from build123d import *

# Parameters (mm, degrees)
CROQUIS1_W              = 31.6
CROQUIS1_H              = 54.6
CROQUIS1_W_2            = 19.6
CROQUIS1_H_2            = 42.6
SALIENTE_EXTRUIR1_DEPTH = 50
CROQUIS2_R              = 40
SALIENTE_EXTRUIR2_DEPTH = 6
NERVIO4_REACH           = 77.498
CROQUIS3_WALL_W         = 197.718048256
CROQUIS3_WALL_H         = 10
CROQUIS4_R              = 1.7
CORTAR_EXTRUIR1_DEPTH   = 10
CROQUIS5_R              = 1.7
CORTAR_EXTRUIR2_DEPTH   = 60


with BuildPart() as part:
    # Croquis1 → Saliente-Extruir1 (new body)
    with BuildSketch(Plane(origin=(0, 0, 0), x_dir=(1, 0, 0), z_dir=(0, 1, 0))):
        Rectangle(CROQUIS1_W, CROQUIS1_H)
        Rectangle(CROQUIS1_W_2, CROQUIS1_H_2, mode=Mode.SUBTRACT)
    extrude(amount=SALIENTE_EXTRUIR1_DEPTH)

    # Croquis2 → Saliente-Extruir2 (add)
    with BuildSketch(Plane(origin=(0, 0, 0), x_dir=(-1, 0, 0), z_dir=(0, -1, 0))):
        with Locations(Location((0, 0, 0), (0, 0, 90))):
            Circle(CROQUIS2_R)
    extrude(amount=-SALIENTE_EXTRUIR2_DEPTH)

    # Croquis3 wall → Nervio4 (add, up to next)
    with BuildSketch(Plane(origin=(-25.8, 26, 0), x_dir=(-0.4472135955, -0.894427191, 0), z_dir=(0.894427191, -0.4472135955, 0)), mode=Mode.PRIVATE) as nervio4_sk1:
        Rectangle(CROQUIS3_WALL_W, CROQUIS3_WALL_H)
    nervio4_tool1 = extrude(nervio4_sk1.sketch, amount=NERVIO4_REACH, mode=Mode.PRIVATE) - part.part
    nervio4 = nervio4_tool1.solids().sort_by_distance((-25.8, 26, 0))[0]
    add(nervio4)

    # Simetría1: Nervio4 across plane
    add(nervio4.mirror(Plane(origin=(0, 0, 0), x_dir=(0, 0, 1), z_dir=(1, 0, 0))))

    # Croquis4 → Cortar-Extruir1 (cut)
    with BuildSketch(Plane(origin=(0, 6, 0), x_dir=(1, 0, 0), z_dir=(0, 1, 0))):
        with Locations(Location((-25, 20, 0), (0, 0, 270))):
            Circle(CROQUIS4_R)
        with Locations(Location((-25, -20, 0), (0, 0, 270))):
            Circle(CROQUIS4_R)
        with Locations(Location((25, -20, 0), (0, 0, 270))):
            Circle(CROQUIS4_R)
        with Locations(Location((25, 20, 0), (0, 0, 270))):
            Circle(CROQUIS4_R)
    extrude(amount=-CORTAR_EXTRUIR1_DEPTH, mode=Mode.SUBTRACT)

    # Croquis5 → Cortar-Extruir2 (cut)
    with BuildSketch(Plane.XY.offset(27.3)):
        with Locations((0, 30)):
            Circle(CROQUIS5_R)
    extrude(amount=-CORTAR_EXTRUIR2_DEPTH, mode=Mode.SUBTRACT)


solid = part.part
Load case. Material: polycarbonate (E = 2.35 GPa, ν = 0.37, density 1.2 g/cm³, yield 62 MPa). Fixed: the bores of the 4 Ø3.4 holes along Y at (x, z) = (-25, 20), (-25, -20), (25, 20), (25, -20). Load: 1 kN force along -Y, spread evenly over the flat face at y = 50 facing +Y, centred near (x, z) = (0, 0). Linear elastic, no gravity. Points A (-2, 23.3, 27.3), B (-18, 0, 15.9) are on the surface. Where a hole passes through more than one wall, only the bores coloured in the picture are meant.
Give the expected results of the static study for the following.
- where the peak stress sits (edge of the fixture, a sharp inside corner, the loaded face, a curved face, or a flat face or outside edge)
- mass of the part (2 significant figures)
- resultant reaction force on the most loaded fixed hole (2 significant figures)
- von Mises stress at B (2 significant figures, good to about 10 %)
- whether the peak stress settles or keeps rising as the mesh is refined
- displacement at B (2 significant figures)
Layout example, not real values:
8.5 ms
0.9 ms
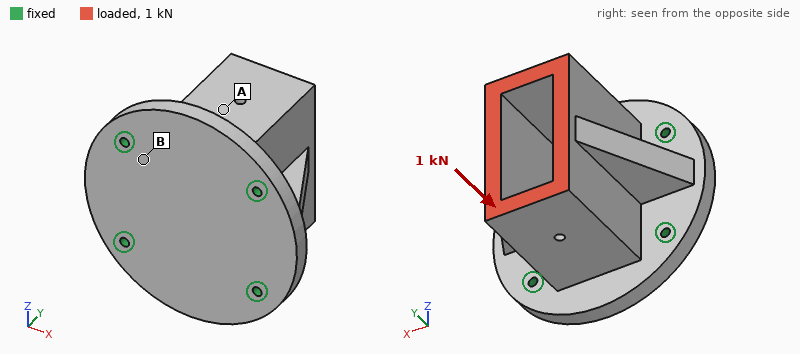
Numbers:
edge of the fixture
92 g
260 N
2.2 MPa
keeps rising
0.052 mm
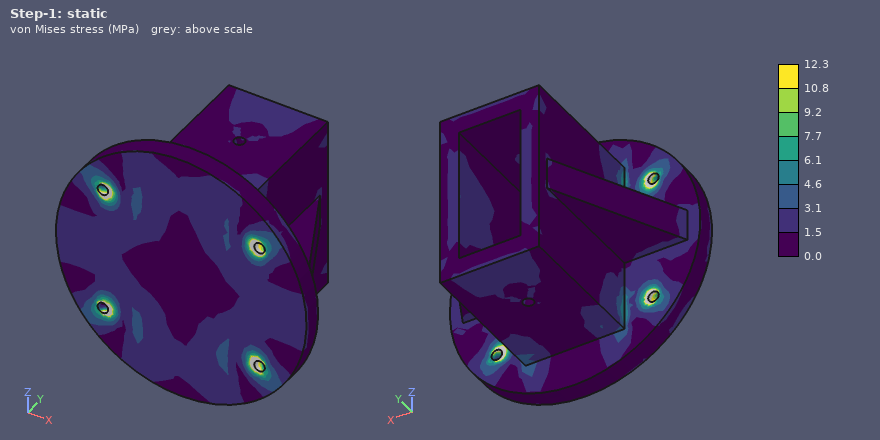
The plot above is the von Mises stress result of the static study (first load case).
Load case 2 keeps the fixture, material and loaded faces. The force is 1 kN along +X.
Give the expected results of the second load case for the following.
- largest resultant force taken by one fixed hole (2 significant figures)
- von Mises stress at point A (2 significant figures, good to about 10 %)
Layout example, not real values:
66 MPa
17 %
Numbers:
550 N
4.3 MPa
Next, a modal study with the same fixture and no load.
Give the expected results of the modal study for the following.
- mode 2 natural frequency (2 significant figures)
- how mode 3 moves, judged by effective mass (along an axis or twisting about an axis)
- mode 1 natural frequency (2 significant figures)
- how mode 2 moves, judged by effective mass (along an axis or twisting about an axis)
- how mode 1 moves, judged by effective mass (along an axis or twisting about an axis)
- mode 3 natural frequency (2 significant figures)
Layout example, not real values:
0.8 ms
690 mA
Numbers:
1600 Hz
along Y
1300 Hz
along X
along Z
1900 Hz
